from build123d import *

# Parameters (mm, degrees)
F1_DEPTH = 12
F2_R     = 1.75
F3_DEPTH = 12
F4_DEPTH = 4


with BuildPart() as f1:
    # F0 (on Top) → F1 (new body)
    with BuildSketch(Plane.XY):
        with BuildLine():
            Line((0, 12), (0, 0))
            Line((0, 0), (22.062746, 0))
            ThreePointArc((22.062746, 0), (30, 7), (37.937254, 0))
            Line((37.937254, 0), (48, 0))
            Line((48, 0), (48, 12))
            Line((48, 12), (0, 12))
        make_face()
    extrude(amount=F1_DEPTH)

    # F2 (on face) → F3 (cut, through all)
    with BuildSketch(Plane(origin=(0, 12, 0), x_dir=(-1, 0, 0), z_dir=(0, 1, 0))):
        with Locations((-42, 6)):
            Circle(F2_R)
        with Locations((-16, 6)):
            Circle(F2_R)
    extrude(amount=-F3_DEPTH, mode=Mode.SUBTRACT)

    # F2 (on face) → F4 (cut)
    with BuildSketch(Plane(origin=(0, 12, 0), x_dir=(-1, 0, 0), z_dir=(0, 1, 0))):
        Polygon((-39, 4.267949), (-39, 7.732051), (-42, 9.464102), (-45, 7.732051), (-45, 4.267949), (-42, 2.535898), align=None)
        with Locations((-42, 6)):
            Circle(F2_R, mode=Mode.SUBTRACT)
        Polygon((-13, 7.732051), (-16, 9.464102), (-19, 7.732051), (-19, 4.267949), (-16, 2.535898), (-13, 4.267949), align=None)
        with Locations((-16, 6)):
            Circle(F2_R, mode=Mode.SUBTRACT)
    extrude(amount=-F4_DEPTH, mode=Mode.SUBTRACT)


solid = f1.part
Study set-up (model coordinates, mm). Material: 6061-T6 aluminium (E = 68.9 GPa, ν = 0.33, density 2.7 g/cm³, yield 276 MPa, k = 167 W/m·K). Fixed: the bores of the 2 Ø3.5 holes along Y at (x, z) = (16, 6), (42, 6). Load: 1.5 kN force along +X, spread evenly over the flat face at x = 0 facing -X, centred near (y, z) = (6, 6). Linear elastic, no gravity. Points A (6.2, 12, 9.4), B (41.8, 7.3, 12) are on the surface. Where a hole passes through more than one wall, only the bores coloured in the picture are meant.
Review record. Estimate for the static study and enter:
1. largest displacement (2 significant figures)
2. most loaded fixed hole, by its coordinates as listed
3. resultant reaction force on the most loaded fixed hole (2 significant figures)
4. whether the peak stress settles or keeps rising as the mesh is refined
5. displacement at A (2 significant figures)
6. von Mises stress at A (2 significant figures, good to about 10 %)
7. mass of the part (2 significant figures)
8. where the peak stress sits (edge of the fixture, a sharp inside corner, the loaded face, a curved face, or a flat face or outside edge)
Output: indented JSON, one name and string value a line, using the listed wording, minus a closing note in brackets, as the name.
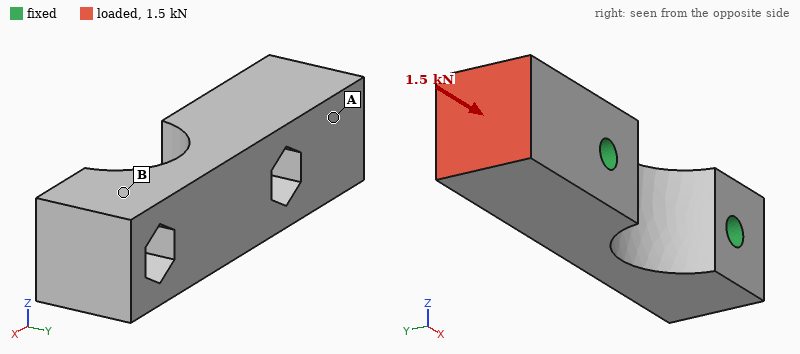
{
  "largest displacement": "5.4 µm",
  "most loaded fixed hole, by its coordinates as listed": "(16, 6)",
  "resultant reaction force on the most loaded fixed hole": "1.4 kN",
  "whether the peak stress settles or keeps rising as the mesh is refined": "keeps rising",
  "displacement at A": "4.0 µm",
  "von Mises stress at A": "9.8 MPa",
  "mass of the part": "15 g",
  "where the peak stress sits": "edge of the fixture"
}
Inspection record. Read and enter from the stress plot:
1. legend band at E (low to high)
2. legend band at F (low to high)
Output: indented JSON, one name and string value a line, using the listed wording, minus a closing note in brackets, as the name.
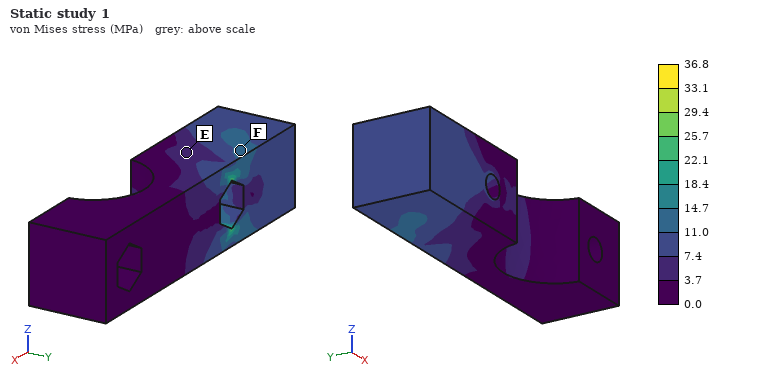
{
  "legend band at E": "3.7 to 7.4 MPa",
  "legend band at F": "11.0 to 14.7 MPa"
}
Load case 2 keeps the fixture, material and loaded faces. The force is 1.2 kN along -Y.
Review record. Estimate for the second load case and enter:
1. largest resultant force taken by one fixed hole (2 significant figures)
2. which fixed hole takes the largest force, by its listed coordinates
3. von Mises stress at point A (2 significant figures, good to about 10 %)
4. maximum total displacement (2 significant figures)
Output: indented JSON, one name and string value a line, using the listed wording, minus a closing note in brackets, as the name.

{
  "largest resultant force taken by one fixed hole": "1.5 kN",
  "which fixed hole takes the largest force, by its listed coordinates": "(16, 6)",
  "von Mises stress at point A": "25 MPa",
  "maximum total displacement": "36 µm"
}
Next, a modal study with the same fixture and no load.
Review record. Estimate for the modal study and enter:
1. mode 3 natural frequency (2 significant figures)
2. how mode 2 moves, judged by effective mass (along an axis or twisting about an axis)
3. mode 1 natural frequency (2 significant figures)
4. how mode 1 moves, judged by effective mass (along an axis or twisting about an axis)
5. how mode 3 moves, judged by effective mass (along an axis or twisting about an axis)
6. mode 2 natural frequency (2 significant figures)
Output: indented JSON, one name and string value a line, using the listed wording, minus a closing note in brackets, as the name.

{
  "mode 3 natural frequency": "32 kHz",
  "how mode 2 moves, judged by effective mass": "along Y",
  "mode 1 natural frequency": "19 kHz",
  "how mode 1 moves, judged by effective mass": "along Z",
  "how mode 3 moves, judged by effective mass": "along Z",
  "mode 2 natural frequency": "21 kHz"
}
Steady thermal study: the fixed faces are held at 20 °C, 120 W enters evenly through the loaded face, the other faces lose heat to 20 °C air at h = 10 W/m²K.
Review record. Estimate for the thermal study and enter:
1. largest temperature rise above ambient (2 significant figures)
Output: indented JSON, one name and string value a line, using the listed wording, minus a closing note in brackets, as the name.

{
  "largest temperature rise above ambient": "87 K"
}
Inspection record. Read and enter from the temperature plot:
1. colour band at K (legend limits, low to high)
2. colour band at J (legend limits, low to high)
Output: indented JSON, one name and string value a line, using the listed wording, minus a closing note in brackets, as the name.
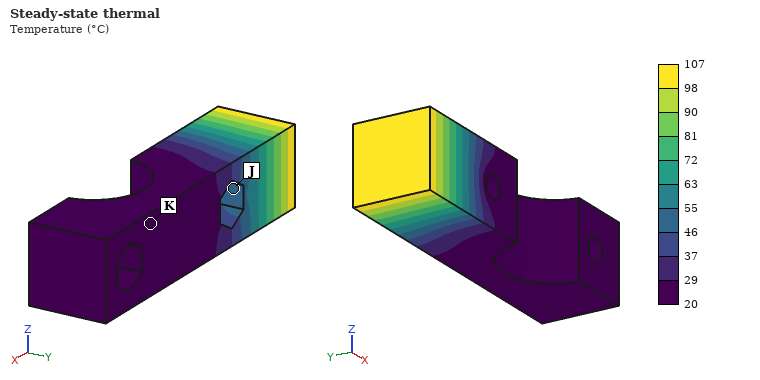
{
  "colour band at K": "20 to 29 °C",
  "colour band at J": "46 to 55 °C"
}
